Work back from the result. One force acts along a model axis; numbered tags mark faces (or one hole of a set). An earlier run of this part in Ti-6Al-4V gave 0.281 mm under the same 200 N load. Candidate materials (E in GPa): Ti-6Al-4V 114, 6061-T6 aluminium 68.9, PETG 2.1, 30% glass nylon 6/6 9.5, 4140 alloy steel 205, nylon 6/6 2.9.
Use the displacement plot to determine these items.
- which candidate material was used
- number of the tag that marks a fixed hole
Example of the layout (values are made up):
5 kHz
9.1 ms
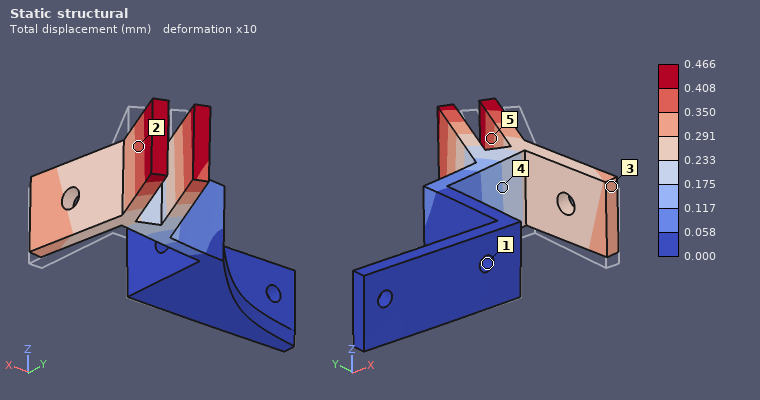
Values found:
6061-T6 aluminium
1
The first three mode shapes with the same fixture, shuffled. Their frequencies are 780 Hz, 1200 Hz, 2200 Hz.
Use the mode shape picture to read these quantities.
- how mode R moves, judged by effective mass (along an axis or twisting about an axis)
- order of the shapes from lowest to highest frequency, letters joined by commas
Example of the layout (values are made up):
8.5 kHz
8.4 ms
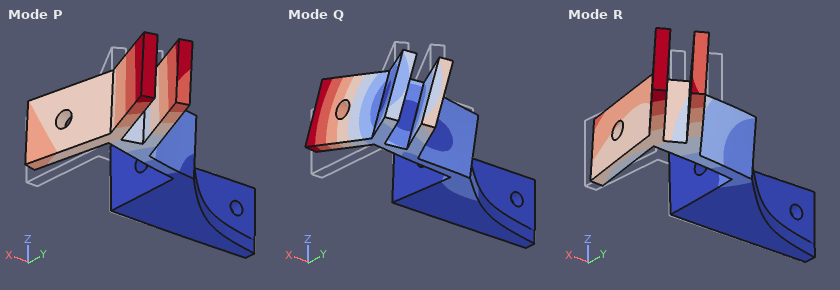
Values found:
along Z
P, R, Q
